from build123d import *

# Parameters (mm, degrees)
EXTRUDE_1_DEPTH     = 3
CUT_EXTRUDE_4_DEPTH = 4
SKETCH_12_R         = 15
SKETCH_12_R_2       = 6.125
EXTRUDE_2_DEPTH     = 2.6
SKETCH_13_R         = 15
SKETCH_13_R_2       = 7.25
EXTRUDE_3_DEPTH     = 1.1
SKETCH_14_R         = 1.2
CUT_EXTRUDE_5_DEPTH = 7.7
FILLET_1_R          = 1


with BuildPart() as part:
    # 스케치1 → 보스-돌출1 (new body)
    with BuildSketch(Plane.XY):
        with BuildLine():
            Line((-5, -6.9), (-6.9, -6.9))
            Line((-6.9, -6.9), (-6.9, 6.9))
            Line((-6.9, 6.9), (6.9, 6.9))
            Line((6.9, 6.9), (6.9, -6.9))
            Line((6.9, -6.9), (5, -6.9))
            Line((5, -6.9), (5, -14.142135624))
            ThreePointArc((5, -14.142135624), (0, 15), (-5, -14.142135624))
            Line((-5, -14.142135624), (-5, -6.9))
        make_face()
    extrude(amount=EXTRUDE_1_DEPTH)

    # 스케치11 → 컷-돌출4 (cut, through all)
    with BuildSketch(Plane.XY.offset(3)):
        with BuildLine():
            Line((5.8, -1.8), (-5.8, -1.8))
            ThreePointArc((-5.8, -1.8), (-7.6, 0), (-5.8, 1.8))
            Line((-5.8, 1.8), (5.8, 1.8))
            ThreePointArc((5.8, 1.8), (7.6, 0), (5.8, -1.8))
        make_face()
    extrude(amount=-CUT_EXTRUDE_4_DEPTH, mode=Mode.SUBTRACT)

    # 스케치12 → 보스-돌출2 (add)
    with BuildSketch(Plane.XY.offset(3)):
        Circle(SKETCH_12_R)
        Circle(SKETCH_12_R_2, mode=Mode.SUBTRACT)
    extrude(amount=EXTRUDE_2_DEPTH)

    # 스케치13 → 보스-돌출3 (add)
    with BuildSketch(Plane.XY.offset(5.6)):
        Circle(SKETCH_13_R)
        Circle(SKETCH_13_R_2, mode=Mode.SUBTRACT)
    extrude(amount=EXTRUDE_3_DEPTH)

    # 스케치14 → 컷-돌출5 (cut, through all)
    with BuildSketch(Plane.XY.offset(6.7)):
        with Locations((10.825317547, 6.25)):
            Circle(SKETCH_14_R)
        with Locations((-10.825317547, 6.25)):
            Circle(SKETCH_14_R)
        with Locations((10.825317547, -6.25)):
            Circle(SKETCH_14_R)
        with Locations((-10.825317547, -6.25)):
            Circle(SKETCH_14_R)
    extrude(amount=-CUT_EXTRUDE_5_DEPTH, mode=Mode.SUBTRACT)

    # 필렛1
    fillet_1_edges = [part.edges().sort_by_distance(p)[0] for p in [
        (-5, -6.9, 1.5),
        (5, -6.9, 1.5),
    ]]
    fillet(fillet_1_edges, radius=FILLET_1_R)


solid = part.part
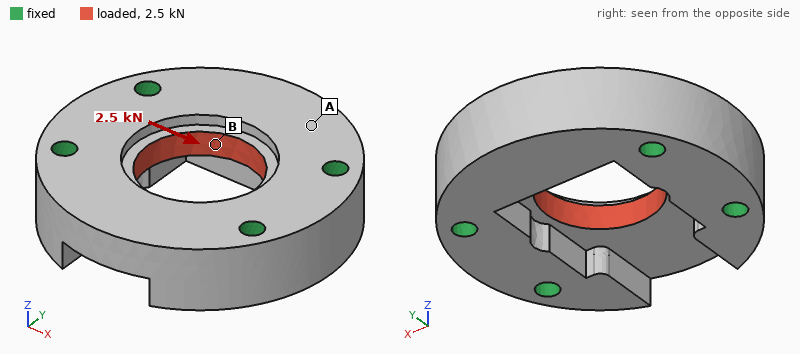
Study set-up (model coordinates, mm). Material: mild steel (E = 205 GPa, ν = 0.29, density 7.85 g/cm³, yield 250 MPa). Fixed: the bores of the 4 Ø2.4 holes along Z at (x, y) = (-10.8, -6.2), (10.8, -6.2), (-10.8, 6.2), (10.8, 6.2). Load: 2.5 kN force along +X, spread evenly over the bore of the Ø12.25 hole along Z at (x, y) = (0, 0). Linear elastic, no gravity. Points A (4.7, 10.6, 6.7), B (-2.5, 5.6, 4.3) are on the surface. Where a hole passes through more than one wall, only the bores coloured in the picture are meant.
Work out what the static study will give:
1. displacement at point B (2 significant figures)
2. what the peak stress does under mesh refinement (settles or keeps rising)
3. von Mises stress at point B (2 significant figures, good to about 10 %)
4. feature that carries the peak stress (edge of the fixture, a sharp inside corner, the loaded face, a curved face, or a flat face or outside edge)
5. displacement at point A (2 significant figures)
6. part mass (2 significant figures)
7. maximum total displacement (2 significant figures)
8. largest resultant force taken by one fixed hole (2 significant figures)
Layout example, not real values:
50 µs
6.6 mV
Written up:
0.82 µm
keeps rising
39 MPa
edge of the fixture
0.33 µm
26 g
1.0 µm
630 N
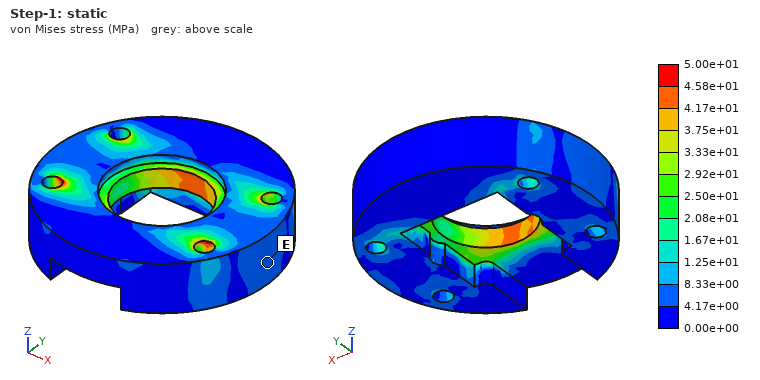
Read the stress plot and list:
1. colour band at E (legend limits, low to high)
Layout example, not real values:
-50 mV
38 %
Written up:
4.17e+00 to 8.33e+00 MPa
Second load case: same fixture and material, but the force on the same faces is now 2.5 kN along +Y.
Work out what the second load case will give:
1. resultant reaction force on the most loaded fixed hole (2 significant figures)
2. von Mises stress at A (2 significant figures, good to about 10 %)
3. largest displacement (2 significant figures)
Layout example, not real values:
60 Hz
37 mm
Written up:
640 N
14 MPa
1.9 µm
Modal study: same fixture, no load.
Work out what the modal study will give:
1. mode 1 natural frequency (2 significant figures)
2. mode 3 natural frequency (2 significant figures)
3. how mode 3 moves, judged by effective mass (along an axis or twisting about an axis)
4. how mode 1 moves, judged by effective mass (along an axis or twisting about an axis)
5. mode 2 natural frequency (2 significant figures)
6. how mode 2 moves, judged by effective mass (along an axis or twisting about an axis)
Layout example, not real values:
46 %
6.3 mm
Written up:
37 kHz
62 kHz
along Y
along Z
41 kHz
along Z
